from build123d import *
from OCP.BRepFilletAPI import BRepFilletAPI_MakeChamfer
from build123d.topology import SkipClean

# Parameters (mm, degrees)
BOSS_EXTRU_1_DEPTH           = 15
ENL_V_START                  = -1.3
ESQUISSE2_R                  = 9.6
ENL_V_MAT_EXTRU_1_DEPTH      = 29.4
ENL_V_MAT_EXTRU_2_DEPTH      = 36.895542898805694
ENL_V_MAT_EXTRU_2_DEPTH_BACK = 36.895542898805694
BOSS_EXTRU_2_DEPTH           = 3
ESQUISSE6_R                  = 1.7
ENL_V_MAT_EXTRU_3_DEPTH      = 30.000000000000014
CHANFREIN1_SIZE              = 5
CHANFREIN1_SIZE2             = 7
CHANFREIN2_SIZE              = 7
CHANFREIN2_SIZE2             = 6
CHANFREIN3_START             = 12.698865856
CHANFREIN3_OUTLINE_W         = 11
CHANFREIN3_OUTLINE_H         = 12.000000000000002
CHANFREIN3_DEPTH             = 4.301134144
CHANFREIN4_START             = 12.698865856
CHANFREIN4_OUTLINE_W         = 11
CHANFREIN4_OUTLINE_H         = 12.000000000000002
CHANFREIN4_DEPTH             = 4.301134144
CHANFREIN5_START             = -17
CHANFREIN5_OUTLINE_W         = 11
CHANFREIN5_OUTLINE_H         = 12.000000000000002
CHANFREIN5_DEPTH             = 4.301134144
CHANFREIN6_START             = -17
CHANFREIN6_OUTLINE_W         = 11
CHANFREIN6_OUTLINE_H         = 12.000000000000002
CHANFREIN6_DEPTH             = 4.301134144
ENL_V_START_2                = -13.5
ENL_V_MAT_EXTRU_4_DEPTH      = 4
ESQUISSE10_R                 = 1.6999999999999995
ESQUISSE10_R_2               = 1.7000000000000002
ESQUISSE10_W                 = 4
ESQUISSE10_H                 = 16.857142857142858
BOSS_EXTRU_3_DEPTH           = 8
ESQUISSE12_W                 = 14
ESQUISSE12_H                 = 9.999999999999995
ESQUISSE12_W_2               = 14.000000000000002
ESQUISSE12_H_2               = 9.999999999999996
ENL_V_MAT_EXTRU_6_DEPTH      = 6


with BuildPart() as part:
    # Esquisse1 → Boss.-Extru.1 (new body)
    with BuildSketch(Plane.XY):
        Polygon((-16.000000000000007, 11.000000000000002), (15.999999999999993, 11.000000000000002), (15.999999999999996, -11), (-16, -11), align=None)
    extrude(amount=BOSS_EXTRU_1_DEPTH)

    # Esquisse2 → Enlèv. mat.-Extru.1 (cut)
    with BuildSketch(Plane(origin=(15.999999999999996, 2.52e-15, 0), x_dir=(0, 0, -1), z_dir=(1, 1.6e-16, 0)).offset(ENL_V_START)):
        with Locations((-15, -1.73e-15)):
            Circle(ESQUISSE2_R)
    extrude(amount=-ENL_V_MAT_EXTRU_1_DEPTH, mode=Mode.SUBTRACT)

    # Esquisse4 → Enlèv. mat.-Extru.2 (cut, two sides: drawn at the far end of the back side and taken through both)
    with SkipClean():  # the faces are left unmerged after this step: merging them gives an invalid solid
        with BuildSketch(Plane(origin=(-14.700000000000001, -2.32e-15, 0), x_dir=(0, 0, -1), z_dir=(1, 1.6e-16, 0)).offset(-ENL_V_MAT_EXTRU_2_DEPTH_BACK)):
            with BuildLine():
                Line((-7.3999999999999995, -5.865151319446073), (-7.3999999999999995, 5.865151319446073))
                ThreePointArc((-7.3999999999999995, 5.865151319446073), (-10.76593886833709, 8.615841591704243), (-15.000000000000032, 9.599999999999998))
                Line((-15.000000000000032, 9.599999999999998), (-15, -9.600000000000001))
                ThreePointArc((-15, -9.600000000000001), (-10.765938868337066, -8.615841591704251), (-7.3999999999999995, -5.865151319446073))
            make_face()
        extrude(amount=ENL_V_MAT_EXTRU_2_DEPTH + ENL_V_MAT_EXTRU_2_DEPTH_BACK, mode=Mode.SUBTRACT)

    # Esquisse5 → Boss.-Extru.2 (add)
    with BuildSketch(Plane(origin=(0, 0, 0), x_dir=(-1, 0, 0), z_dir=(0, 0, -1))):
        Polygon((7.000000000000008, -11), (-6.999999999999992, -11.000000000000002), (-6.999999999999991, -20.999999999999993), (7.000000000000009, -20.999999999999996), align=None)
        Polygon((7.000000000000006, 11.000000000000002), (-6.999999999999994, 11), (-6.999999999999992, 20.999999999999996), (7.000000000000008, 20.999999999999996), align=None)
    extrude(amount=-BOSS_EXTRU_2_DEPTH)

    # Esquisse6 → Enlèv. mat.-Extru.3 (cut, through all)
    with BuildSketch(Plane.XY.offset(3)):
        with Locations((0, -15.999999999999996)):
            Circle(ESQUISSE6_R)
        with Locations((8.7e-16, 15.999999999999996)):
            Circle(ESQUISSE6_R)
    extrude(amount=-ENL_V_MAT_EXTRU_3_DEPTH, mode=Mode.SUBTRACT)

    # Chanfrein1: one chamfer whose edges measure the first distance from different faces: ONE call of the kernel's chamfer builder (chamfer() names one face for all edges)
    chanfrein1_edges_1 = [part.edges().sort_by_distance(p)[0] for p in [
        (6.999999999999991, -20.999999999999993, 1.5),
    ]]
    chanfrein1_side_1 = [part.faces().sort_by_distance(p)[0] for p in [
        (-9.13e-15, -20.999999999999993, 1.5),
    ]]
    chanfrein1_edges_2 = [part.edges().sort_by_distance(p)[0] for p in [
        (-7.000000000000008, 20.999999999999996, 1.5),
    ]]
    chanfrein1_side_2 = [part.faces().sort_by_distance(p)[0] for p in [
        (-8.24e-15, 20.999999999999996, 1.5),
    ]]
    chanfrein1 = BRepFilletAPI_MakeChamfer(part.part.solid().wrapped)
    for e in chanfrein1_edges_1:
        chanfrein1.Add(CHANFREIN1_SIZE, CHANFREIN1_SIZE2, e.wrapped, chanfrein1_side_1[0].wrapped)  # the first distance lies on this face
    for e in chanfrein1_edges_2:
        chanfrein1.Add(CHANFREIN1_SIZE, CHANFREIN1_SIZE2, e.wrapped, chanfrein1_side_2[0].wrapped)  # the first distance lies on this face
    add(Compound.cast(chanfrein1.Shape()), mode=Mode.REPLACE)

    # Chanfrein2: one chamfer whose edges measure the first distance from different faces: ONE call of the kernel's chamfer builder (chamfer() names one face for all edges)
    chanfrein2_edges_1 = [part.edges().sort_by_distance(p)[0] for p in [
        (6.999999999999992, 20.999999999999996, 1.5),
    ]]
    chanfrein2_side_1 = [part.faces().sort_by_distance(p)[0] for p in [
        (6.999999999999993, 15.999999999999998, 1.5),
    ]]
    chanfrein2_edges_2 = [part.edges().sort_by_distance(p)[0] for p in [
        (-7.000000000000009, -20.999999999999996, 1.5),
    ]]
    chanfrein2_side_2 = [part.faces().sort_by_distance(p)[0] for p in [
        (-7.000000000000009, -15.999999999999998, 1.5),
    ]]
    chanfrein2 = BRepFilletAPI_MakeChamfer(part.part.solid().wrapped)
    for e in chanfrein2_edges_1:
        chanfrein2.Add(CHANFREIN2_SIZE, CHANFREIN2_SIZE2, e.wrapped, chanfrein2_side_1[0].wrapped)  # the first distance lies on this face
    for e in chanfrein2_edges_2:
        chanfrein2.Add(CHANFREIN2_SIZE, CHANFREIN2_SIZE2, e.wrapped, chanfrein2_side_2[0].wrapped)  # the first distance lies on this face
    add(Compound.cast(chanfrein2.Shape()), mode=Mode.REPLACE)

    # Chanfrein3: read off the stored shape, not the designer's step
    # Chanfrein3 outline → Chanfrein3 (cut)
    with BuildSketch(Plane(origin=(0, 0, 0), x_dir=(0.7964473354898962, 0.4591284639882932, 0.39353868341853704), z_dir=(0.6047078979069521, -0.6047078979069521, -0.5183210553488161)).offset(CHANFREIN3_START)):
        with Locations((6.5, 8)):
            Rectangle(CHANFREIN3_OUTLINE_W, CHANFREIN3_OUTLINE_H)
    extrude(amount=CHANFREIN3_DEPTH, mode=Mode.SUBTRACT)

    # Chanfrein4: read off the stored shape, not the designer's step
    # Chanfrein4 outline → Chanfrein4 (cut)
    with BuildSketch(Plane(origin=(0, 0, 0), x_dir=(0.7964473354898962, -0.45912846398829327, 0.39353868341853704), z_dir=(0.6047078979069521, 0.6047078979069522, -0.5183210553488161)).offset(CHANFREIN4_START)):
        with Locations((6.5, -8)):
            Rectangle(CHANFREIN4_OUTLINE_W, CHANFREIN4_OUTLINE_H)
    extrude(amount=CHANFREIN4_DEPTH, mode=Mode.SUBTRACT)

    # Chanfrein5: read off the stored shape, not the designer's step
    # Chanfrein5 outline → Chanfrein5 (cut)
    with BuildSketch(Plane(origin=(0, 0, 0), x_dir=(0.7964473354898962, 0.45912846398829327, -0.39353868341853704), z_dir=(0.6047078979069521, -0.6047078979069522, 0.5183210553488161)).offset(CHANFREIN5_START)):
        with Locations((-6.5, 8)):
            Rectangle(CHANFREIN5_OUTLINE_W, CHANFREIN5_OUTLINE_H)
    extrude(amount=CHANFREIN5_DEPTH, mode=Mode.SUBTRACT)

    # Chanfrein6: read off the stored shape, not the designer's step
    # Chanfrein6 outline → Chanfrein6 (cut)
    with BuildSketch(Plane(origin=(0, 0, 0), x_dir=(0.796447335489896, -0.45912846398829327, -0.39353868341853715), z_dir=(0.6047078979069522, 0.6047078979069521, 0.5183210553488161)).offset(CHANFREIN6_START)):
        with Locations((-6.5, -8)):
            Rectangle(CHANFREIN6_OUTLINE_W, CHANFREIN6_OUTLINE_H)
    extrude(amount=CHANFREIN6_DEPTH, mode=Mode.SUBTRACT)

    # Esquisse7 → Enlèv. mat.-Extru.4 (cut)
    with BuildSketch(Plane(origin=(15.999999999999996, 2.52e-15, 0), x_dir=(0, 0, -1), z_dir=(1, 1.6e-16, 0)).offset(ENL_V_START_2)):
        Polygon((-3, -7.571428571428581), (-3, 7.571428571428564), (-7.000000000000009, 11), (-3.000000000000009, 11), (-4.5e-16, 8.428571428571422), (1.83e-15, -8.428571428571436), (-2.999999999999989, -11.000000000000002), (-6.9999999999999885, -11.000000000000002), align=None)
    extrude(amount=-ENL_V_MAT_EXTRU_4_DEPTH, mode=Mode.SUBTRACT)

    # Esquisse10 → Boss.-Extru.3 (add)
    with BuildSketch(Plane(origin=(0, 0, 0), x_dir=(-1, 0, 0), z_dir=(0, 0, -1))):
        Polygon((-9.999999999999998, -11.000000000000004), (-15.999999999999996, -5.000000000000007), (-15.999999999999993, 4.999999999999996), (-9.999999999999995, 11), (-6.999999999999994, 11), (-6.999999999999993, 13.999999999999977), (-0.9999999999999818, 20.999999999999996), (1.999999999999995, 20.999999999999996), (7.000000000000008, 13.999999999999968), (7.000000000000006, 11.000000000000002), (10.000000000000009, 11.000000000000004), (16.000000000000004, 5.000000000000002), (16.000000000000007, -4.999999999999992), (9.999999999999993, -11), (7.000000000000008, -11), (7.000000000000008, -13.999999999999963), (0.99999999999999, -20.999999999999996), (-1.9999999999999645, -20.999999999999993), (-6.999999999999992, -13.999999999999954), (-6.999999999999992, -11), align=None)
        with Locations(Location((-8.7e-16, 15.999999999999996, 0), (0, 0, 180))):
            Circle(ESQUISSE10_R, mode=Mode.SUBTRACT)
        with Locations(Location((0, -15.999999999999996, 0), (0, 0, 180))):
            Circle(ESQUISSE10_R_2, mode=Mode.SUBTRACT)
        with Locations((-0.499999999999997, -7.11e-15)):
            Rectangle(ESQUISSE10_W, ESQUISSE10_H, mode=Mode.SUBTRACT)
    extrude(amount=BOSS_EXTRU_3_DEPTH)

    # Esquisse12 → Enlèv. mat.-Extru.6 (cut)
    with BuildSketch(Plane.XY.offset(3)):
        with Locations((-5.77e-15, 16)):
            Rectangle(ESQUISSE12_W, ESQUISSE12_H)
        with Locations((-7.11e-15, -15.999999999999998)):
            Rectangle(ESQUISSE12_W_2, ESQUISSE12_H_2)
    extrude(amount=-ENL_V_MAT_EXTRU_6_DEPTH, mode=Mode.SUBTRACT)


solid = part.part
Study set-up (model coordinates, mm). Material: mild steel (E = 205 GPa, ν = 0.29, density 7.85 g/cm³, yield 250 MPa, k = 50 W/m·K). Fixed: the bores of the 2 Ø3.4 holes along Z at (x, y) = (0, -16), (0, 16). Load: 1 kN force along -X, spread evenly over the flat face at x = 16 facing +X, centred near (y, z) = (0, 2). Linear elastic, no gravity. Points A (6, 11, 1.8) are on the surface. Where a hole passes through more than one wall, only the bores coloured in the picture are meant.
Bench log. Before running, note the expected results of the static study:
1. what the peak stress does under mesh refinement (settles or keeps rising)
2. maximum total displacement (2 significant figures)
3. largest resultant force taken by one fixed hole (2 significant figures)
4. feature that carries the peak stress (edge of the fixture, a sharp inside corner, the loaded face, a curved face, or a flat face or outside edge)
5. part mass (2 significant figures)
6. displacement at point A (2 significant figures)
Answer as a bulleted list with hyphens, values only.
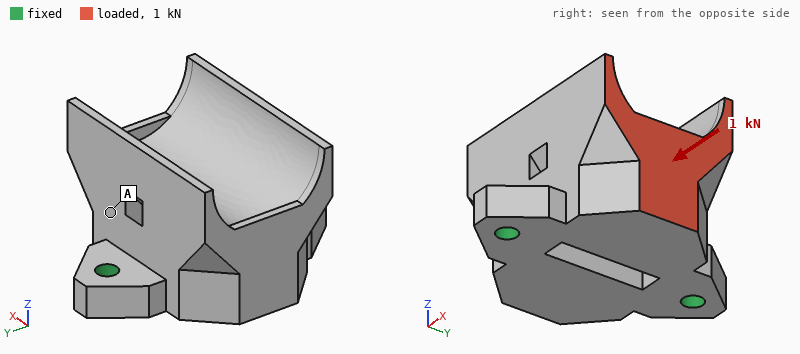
- keeps rising
- 19 µm
- 500 N
- edge of the fixture
- 86 g
- 7.1 µm
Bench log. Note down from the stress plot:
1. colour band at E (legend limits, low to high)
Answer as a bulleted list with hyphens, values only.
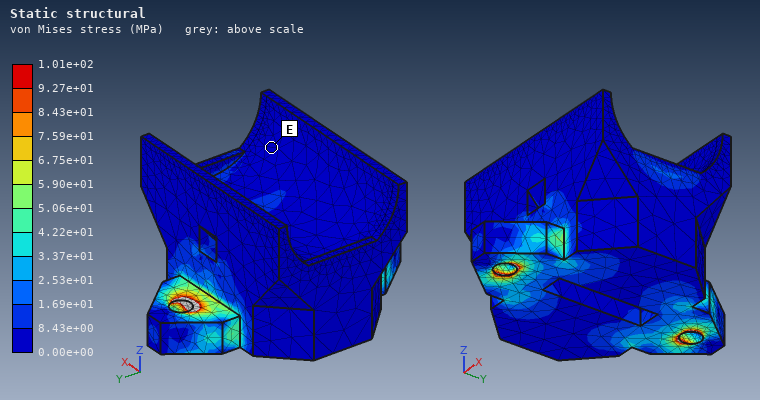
- 0.00e+00 to 8.43e+00 MPa
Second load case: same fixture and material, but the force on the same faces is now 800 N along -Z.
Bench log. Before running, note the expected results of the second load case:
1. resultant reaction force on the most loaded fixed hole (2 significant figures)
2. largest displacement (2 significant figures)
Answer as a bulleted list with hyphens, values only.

- 470 N
- 30 µm
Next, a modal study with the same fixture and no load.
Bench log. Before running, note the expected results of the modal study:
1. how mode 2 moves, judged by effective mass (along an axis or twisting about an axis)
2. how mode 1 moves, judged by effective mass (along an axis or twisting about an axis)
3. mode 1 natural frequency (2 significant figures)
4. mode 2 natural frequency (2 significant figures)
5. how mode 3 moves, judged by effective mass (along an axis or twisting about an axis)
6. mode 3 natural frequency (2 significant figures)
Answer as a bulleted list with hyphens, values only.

- along Z
- along X
- 4900 Hz
- 14 kHz
- along Y
- 16 kHz
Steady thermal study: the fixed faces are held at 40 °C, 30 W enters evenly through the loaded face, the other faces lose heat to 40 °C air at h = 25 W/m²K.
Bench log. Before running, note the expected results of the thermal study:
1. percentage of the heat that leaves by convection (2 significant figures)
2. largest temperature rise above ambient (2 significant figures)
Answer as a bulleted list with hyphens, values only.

- 13 %
- 73 K
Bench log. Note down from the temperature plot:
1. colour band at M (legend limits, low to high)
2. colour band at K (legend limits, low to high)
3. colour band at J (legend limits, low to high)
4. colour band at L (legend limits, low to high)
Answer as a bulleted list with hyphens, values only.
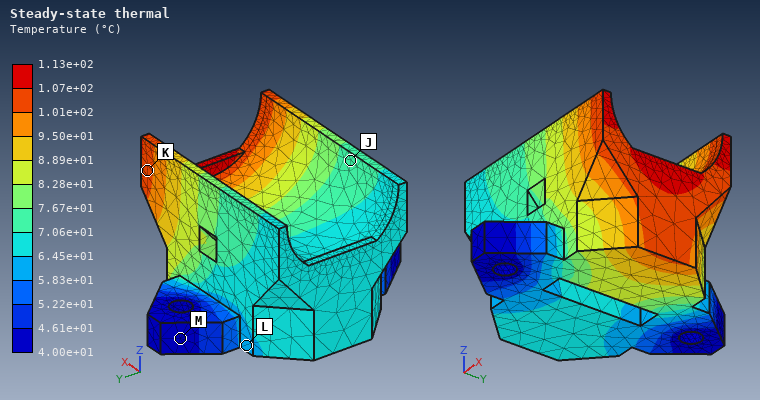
- 4.00e+01 to 4.61e+01 °C
- 1.01e+02 to 1.07e+02 °C
- 7.06e+01 to 7.67e+01 °C
- 5.83e+01 to 6.45e+01 °C
